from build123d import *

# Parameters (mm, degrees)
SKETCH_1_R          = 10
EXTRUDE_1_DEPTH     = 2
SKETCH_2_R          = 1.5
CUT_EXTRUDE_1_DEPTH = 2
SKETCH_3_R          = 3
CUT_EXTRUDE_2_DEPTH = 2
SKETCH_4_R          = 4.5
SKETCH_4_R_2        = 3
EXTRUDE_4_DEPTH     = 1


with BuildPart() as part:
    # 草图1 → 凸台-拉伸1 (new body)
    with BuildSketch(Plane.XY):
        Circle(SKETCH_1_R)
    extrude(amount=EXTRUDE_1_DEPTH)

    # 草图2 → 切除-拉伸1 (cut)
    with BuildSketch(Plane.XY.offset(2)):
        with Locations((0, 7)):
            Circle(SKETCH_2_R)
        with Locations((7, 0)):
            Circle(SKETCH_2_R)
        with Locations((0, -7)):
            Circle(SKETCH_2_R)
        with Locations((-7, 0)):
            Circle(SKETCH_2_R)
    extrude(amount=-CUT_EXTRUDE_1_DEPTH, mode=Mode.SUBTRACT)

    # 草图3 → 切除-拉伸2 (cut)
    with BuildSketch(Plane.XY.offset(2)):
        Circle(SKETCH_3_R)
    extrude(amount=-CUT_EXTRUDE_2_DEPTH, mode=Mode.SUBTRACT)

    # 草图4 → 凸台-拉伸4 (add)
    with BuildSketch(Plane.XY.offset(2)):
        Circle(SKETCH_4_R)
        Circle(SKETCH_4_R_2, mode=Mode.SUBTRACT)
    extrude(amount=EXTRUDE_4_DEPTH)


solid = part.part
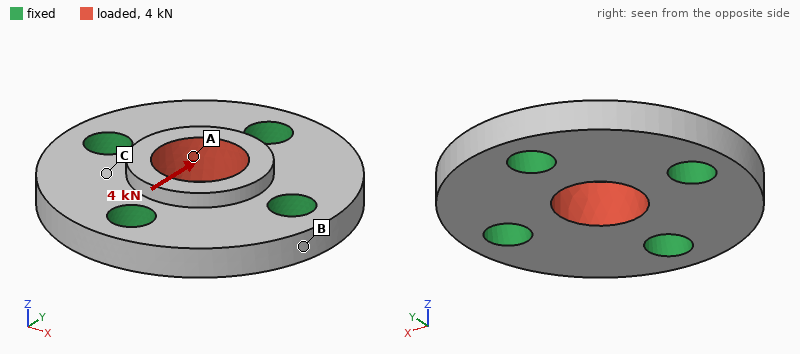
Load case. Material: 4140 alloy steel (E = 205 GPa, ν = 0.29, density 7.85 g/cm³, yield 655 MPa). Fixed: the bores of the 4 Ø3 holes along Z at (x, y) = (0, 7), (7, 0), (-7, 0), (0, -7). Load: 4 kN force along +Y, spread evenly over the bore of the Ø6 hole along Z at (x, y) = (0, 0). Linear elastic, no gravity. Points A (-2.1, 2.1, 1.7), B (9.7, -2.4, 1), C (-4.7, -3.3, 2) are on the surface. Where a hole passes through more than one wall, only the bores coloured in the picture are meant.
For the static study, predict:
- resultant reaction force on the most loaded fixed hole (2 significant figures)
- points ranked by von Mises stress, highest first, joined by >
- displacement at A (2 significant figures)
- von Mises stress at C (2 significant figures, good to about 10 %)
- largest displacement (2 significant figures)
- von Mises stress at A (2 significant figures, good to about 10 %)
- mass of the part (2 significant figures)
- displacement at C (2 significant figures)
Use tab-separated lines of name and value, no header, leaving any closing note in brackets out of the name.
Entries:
resultant reaction force on the most loaded fixed hole	1.2 kN
points ranked by von Mises stress, highest first, joined by >	A > C > B
displacement at A	2.5 µm
von Mises stress at C	53 MPa
largest displacement	3.3 µm
von Mises stress at A	120 MPa
mass of the part	4.3 g
displacement at C	1.2 µm
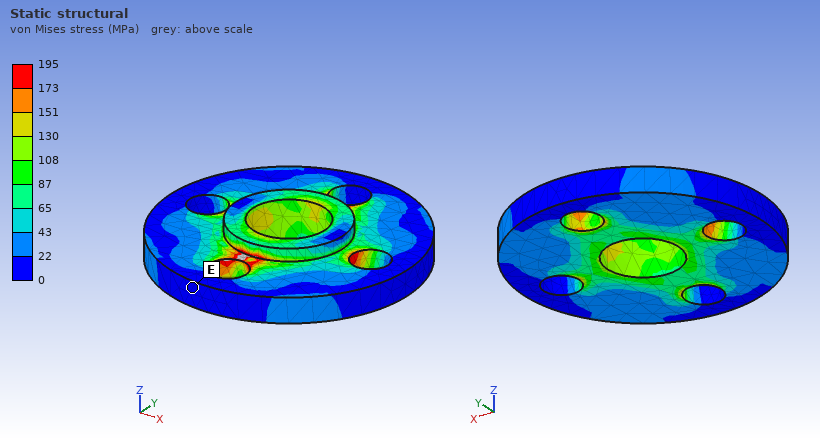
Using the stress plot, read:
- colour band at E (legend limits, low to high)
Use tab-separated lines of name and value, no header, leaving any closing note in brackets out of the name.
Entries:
colour band at E	0 to 22 MPa
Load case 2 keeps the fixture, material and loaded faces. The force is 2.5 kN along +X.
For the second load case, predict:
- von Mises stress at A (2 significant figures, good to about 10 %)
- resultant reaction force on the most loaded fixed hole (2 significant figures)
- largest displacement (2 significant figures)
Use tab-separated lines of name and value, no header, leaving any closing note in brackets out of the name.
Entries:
von Mises stress at A	77 MPa
resultant reaction force on the most loaded fixed hole	770 N
largest displacement	2.1 µm
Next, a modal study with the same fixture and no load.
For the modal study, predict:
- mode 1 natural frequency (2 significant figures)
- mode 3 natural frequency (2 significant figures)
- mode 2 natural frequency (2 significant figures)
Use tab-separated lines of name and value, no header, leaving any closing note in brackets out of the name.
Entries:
mode 1 natural frequency	77 kHz
mode 3 natural frequency	78 kHz
mode 2 natural frequency	78 kHz
